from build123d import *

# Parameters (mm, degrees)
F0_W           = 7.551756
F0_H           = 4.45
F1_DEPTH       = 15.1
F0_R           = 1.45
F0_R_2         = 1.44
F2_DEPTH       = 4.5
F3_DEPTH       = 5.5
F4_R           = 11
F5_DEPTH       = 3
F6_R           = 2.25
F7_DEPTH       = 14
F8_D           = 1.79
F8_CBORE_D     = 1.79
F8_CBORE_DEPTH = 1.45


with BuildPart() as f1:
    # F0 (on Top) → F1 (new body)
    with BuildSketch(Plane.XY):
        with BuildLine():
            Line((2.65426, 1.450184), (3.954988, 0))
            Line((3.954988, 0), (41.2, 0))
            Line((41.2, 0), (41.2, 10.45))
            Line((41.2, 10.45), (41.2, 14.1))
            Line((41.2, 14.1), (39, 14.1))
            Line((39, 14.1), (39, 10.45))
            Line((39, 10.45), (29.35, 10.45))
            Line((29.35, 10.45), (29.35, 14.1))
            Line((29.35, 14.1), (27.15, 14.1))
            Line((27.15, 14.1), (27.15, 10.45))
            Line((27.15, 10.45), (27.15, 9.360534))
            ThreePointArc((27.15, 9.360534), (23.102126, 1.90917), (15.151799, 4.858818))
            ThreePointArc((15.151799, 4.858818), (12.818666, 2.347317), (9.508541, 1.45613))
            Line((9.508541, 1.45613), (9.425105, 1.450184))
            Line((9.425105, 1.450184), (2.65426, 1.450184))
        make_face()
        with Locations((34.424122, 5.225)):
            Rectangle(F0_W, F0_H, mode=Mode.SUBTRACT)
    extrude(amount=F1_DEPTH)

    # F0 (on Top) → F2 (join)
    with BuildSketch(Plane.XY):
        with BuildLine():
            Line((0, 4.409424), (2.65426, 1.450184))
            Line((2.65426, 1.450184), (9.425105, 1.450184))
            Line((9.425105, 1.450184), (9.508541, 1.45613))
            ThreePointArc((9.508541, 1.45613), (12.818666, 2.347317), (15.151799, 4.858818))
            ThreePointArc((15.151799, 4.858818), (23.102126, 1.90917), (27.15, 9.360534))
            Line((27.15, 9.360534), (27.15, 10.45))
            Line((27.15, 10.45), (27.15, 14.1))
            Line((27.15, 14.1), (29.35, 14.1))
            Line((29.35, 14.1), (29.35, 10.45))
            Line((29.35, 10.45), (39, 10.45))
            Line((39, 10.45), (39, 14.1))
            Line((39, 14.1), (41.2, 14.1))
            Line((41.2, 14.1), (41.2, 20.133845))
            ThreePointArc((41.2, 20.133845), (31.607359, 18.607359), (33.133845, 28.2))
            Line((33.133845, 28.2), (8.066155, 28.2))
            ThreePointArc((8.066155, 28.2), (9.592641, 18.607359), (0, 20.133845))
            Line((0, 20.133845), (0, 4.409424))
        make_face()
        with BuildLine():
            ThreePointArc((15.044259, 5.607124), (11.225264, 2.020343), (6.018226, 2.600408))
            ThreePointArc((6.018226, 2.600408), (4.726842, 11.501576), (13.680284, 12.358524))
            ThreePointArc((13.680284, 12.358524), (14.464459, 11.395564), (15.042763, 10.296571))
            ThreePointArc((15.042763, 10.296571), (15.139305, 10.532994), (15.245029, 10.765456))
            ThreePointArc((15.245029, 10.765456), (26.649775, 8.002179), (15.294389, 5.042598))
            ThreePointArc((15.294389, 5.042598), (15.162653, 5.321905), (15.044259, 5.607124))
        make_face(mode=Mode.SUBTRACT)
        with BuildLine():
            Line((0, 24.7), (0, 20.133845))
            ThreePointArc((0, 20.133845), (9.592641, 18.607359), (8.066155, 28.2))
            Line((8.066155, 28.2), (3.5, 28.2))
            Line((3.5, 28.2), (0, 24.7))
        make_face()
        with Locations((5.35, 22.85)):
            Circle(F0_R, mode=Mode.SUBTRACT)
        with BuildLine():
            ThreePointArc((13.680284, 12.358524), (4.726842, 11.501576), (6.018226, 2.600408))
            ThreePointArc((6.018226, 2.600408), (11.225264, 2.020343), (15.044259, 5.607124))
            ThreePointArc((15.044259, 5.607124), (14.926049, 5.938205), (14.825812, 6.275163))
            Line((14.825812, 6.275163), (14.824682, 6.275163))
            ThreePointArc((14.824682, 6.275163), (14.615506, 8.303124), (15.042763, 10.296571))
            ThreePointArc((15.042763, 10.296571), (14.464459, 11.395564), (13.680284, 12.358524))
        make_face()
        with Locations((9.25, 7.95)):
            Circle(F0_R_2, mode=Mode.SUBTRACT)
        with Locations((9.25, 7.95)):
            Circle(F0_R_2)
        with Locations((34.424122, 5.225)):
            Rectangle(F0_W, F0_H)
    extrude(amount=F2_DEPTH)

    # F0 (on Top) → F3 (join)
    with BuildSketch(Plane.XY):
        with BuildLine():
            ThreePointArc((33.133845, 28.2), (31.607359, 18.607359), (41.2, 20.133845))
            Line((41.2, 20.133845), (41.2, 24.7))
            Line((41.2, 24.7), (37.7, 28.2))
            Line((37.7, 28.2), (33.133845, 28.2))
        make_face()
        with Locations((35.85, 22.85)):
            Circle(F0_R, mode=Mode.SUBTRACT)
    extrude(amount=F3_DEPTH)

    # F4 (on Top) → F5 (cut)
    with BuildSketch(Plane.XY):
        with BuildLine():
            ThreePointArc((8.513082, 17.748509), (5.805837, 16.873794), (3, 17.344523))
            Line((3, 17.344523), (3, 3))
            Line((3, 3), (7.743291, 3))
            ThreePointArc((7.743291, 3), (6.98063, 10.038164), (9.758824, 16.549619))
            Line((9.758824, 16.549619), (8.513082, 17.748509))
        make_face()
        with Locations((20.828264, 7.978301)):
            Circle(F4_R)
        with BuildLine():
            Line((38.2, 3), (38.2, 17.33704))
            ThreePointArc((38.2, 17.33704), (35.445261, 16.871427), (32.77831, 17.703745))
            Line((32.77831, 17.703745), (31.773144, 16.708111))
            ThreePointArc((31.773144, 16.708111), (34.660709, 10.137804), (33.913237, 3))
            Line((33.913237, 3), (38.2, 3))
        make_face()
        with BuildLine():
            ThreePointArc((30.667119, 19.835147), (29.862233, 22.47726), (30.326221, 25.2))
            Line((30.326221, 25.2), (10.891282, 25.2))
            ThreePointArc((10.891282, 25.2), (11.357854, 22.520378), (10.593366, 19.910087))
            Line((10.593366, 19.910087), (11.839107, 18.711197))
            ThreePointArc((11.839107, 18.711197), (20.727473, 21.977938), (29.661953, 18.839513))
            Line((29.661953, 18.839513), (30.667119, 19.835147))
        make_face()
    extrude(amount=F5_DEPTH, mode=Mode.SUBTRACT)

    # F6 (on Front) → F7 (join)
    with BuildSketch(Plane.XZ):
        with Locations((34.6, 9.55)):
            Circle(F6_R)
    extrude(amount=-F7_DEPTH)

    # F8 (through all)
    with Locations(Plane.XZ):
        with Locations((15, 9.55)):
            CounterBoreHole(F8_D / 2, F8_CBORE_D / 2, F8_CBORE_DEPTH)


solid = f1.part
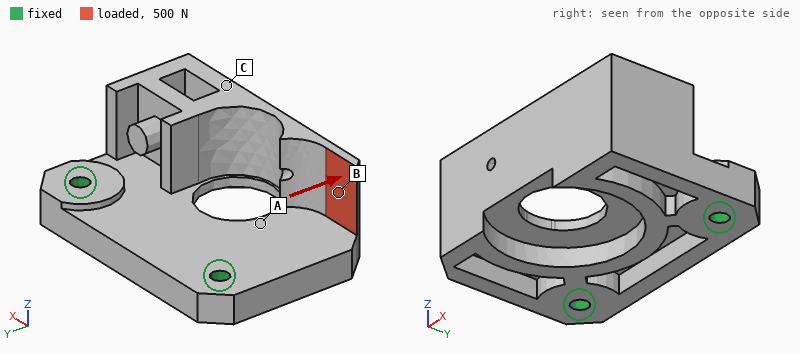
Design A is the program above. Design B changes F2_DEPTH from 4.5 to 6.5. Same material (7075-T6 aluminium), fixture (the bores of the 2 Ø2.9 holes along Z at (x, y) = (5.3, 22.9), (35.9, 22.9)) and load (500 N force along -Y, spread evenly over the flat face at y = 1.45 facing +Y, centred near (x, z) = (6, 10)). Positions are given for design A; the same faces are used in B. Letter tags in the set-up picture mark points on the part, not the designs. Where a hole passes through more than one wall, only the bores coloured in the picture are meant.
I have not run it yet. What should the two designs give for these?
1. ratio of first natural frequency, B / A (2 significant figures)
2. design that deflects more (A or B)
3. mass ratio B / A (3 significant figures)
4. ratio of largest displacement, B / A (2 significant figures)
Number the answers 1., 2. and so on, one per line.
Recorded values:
1. 1.4
2. A
3. 1.27
4. 0.64
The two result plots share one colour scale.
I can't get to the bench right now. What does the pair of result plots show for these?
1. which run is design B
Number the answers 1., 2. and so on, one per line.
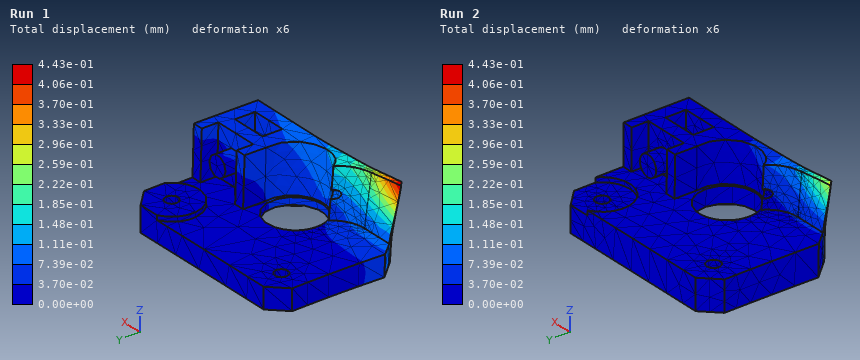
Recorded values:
1. Run 2
